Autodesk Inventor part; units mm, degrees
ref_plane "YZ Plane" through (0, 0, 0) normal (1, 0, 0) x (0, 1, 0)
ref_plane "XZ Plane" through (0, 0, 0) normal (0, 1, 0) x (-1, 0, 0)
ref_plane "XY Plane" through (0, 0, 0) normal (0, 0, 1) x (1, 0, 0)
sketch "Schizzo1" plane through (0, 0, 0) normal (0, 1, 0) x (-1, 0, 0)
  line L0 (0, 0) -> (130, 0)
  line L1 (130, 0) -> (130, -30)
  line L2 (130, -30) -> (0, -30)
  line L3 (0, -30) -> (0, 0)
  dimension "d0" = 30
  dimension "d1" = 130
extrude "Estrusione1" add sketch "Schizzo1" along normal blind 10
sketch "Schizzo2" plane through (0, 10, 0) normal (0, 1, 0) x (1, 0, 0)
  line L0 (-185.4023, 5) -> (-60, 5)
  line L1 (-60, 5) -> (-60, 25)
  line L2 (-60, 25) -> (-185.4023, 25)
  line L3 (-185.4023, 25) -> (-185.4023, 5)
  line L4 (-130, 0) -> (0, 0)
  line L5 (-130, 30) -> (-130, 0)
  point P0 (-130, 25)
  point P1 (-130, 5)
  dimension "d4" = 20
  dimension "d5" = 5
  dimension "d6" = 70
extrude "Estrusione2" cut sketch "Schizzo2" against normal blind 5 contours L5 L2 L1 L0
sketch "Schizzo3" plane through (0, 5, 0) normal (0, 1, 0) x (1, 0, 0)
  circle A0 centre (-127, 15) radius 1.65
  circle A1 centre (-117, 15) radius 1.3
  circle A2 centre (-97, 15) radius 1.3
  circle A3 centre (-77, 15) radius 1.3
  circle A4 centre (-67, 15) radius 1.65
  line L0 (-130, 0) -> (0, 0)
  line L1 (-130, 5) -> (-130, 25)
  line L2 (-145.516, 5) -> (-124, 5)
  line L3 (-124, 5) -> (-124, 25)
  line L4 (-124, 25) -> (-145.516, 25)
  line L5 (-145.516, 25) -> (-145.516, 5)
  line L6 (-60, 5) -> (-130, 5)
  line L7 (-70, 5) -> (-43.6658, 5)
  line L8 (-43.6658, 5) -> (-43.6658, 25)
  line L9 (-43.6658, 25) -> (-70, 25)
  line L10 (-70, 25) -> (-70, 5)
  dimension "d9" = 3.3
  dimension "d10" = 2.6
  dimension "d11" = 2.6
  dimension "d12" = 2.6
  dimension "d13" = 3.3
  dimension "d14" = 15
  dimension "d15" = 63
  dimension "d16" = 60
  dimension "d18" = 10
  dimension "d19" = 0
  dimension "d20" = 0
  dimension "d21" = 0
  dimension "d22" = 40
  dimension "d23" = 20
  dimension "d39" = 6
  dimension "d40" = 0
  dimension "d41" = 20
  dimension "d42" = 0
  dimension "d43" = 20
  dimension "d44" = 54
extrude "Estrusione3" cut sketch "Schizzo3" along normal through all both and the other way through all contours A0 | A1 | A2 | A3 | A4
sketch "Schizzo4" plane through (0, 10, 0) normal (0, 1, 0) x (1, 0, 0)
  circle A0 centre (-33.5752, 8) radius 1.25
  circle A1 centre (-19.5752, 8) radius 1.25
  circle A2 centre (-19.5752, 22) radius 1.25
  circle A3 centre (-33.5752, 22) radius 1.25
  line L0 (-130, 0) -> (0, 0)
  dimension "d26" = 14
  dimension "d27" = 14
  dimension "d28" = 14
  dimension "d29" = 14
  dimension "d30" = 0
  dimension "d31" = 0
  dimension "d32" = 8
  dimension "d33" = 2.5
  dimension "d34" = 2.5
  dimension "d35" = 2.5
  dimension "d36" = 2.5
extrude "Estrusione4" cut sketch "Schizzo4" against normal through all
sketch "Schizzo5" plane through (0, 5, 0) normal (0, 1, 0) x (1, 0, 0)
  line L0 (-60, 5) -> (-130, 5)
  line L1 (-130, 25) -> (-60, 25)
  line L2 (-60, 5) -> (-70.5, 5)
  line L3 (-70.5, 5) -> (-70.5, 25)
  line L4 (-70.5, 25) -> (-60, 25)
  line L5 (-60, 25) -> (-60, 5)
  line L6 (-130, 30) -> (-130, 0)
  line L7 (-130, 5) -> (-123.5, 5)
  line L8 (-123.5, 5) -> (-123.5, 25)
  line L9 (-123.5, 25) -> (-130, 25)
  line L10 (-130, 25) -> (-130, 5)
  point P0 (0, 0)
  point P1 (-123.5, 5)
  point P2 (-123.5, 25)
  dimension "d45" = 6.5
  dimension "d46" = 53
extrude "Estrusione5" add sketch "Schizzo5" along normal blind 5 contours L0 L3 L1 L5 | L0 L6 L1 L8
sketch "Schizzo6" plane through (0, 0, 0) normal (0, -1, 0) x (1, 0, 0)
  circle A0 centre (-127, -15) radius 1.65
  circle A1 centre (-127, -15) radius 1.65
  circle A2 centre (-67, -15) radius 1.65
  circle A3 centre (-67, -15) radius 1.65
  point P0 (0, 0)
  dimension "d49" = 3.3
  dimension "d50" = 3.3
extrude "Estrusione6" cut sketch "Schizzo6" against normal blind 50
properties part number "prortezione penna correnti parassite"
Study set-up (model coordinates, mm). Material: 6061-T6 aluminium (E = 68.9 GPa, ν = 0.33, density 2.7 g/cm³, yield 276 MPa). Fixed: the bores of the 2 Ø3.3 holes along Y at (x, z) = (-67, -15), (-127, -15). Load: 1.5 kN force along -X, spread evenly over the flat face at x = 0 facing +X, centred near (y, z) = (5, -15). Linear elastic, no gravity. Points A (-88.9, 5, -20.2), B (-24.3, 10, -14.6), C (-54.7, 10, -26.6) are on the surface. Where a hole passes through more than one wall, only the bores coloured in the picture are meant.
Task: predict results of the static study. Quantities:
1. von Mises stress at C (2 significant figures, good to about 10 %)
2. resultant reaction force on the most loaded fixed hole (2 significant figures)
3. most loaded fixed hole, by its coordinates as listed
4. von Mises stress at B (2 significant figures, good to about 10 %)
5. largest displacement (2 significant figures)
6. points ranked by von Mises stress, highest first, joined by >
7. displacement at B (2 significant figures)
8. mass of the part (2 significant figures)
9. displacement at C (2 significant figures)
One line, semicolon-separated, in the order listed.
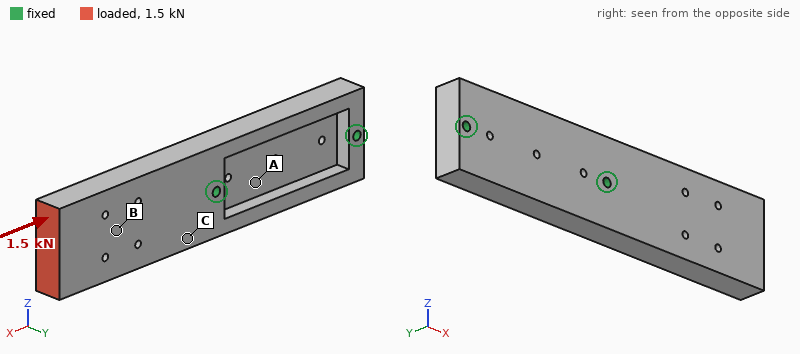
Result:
4.1 MPa; 1.3 kN; (-67, -15); 5.6 MPa; 6.0 µm; B > C > A; 4.2 µm; 90 g; 2.0 µm
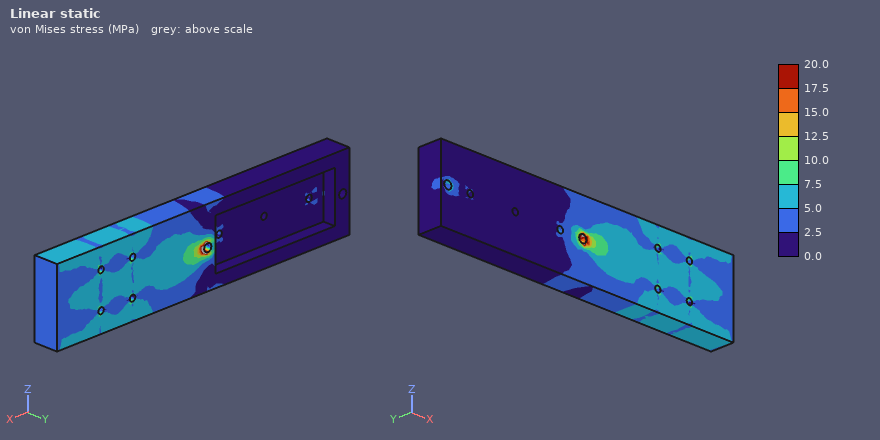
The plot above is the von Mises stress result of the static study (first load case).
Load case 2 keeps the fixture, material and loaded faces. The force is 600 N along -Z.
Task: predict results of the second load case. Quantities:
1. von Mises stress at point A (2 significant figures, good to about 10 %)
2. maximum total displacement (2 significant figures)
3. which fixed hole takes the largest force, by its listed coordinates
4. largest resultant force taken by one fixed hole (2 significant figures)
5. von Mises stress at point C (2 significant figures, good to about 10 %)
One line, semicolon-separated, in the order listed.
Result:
11 MPa; 97 µm; (-67, -15); 1.2 kN; 17 MPa
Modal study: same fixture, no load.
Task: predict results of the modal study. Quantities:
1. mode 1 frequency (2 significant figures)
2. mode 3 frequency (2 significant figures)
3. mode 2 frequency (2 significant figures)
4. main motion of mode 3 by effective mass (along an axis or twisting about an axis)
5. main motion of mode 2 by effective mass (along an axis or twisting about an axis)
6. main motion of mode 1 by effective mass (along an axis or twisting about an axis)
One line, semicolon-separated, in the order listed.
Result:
1600 Hz; 5900 Hz; 3100 Hz; twisting about X; along Z; along Y
